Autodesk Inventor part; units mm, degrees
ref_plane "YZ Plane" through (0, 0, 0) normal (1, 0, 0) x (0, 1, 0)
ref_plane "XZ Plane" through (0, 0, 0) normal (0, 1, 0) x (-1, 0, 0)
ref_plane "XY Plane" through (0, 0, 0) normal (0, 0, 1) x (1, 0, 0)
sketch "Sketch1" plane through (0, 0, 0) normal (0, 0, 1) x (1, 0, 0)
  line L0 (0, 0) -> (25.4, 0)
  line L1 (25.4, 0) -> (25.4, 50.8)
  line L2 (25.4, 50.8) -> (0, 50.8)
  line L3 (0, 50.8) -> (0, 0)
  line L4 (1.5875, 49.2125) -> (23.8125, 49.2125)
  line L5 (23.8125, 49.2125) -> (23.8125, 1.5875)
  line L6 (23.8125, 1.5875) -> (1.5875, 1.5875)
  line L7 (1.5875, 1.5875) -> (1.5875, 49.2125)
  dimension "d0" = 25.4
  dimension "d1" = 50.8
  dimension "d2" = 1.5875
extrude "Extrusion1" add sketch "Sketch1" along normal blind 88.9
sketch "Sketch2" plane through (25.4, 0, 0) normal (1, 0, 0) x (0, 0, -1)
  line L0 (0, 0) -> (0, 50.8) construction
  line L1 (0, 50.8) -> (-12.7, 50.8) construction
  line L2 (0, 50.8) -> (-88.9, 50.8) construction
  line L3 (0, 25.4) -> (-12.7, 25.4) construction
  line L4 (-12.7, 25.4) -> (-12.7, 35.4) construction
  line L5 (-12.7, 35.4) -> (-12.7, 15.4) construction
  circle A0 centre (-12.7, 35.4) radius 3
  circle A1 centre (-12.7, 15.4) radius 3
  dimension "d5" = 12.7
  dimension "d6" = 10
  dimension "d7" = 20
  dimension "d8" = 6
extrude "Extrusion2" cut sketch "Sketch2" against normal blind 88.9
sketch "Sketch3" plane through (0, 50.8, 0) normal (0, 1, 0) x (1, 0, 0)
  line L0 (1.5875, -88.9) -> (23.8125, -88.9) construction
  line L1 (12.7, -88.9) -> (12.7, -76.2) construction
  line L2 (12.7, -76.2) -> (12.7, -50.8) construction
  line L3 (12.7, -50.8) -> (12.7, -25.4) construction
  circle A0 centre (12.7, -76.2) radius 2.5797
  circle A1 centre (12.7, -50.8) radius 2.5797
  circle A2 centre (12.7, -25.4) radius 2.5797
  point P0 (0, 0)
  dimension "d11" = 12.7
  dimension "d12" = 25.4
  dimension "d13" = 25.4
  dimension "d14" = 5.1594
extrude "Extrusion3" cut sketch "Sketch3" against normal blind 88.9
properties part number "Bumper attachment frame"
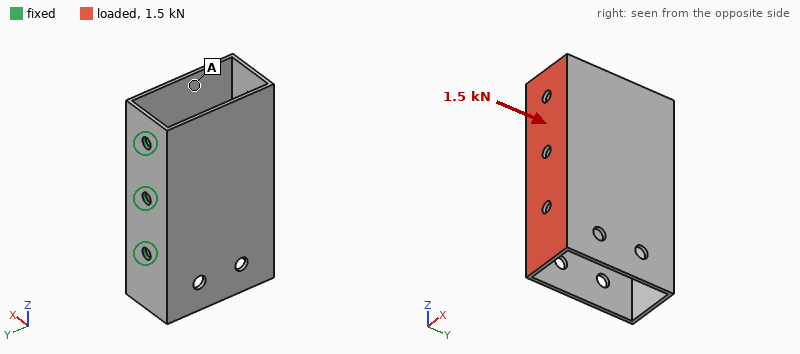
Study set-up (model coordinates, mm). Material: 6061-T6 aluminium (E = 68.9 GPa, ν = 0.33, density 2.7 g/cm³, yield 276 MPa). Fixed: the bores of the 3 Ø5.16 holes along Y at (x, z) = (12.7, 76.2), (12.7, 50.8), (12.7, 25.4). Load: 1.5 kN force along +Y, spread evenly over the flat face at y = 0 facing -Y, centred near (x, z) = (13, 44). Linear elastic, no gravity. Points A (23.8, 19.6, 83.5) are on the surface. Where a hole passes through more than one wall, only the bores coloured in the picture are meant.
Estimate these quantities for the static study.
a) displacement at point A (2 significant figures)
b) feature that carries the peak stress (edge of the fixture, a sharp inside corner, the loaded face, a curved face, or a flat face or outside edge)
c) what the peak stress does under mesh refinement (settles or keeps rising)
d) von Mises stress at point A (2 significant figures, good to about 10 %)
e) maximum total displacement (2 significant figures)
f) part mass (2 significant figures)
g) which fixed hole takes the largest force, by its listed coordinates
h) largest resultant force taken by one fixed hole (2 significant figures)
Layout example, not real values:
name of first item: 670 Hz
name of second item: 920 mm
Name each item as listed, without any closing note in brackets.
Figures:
displacement at point A: 0.17 mm
feature that carries the peak stress: edge of the fixture
what the peak stress does under mesh refinement: keeps rising
von Mises stress at point A: 32 MPa
maximum total displacement: 0.29 mm
part mass: 55 g
which fixed hole takes the largest force, by its listed coordinates: (12.7, 25.4)
largest resultant force taken by one fixed hole: 690 N
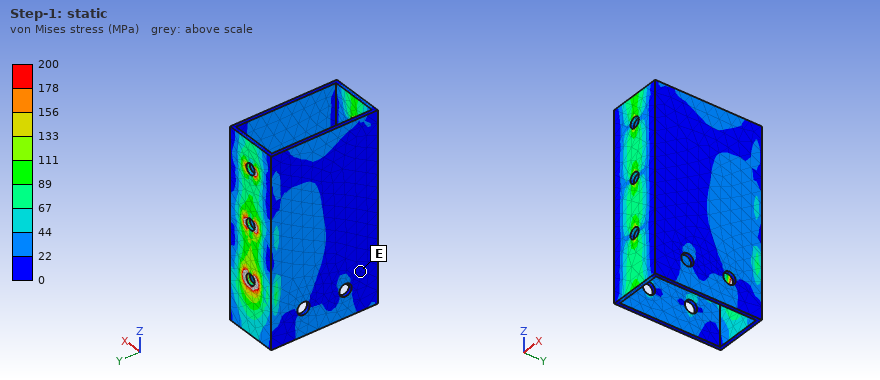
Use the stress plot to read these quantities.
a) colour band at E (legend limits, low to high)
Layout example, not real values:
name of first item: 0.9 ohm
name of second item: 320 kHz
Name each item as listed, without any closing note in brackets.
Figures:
colour band at E: 0 to 22 MPa
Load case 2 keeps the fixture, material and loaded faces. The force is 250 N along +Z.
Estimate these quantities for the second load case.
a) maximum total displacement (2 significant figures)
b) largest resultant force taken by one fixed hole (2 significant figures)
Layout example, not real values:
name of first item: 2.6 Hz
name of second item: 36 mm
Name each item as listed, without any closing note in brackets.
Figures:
maximum total displacement: 0.13 mm
largest resultant force taken by one fixed hole: 240 N
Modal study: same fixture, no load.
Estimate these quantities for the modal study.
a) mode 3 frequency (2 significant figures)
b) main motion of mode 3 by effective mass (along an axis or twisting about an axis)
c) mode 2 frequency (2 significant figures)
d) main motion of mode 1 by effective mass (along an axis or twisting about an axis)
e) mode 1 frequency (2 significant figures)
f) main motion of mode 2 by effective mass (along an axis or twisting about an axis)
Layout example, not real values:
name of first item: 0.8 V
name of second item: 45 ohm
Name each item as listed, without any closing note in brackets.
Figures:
mode 3 frequency: 1400 Hz
main motion of mode 3 by effective mass: along Z
mode 2 frequency: 1300 Hz
main motion of mode 1 by effective mass: along X
mode 1 frequency: 420 Hz
main motion of mode 2 by effective mass: twisting about Y
